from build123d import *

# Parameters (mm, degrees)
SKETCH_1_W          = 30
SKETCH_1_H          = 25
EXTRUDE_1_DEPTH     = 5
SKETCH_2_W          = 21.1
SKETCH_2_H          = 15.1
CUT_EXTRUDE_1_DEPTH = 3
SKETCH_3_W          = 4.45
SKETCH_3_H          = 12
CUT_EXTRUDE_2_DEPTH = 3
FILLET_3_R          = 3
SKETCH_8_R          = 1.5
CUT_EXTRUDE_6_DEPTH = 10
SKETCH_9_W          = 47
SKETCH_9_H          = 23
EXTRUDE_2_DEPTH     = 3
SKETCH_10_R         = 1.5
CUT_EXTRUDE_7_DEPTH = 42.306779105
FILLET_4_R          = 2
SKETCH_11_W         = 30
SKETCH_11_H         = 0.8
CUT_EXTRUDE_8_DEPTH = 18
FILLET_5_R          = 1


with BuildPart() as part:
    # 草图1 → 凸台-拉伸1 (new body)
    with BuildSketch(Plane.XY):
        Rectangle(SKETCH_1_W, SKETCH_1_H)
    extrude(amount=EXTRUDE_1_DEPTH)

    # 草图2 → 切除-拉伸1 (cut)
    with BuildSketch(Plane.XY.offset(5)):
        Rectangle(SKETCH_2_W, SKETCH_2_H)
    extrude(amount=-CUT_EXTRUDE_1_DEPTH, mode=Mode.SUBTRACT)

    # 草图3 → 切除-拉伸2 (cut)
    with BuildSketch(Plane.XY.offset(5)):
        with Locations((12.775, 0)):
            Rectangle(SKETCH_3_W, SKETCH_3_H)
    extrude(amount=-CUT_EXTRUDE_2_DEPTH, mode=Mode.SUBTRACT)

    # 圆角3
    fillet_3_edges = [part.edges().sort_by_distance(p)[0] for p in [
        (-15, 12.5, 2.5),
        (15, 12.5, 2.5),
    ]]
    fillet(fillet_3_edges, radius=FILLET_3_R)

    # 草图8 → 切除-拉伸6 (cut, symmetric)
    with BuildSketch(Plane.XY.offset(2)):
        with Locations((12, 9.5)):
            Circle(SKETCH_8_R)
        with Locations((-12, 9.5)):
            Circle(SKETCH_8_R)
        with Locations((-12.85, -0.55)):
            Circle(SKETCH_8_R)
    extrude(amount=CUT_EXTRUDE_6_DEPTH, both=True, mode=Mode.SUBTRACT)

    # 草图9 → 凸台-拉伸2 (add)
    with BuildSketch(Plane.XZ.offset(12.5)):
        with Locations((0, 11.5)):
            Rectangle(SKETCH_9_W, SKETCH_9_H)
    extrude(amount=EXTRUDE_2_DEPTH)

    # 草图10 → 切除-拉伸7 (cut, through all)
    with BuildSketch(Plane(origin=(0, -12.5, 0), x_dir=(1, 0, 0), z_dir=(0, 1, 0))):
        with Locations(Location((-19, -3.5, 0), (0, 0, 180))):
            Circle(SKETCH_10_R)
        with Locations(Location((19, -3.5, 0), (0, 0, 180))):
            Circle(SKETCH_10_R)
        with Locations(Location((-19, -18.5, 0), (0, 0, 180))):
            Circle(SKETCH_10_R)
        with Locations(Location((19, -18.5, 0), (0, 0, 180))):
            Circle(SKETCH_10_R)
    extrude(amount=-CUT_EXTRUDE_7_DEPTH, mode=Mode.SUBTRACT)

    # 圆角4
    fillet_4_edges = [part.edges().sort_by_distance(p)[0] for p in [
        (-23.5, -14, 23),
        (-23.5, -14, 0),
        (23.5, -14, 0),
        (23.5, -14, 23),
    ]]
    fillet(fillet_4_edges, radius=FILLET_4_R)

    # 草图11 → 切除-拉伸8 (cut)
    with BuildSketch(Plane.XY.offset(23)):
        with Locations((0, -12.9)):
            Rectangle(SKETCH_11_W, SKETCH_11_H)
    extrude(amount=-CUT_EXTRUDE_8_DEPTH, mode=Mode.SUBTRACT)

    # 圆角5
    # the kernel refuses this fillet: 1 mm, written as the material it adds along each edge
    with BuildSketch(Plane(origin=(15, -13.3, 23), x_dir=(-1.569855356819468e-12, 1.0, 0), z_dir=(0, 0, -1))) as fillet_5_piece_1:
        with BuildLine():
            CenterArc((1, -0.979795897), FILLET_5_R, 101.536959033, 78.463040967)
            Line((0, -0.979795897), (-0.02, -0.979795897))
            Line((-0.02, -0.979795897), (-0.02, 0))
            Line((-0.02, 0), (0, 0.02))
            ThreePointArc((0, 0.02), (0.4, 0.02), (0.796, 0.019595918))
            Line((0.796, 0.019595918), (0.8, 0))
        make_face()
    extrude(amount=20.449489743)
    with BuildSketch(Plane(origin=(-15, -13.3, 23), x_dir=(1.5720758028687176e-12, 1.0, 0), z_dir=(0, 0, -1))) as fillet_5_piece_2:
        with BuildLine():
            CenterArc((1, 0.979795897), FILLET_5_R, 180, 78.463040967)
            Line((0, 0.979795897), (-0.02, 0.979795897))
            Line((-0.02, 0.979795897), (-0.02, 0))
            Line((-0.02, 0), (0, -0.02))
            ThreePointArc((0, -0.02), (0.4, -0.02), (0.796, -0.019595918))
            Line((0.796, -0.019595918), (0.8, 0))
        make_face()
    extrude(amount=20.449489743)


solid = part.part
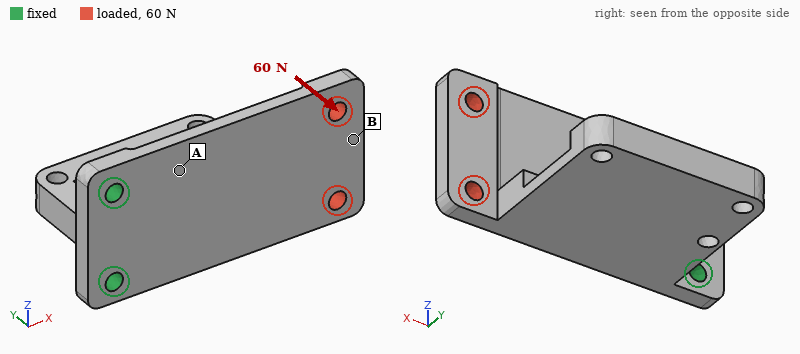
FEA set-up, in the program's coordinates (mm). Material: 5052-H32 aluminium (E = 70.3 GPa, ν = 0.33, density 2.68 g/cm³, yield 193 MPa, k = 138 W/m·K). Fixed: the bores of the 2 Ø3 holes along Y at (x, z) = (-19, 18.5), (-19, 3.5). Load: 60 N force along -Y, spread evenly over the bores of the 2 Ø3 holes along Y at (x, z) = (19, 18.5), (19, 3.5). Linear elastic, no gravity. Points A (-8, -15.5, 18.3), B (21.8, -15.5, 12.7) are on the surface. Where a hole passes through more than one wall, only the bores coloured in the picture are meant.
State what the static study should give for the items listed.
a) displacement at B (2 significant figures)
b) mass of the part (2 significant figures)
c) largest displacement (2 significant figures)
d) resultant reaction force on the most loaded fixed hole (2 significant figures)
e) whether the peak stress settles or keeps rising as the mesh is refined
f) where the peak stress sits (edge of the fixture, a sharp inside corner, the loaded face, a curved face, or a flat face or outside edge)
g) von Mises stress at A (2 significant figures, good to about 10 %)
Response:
0.24 mm
14 g
0.26 mm
36 N
keeps rising
a sharp inside corner
27 MPa
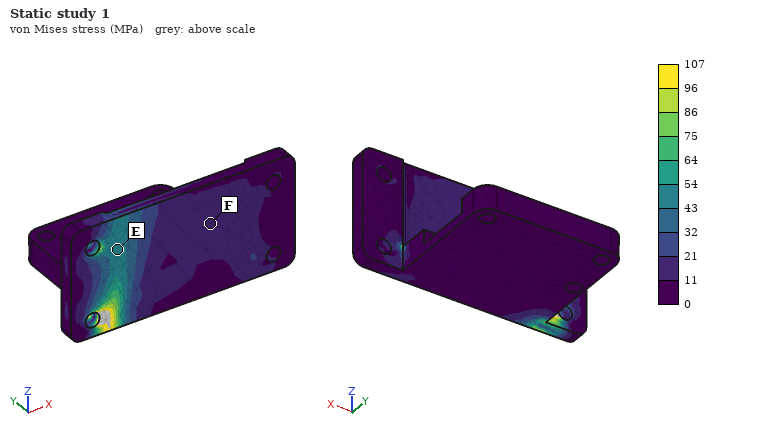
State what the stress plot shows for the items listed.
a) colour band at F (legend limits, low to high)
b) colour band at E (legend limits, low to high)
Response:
11 to 21 MPa
43 to 54 MPa
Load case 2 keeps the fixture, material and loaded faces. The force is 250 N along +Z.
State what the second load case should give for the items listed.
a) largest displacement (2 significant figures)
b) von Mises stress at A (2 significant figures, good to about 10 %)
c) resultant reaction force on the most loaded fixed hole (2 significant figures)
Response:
54 µm
15 MPa
590 N
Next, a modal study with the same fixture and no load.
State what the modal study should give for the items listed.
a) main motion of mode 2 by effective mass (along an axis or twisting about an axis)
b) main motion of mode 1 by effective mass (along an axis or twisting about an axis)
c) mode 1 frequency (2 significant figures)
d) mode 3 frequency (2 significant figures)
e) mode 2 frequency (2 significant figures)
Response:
along Z
along Y
1100 Hz
5100 Hz
2100 Hz
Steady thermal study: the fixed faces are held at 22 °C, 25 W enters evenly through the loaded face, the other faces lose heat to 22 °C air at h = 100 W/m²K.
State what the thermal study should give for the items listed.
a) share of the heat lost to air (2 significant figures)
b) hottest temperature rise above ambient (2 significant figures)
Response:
47 %
72 K
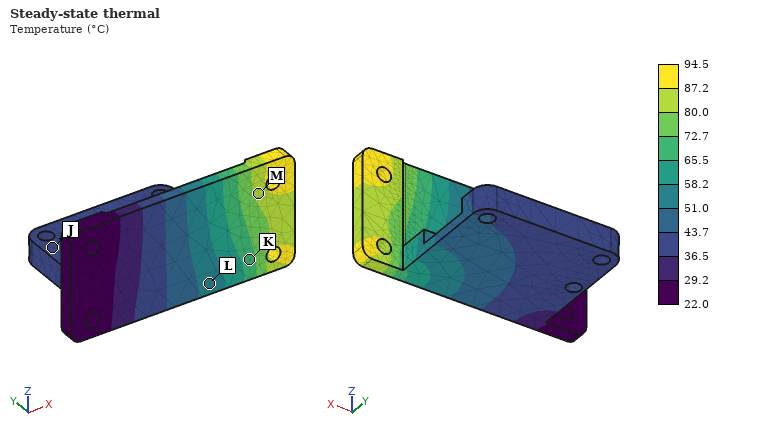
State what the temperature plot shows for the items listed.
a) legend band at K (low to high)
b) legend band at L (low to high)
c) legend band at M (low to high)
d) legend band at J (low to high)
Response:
65.5 to 72.7 °C
51.0 to 58.2 °C
80.0 to 87.2 °C
36.5 to 43.7 °C
